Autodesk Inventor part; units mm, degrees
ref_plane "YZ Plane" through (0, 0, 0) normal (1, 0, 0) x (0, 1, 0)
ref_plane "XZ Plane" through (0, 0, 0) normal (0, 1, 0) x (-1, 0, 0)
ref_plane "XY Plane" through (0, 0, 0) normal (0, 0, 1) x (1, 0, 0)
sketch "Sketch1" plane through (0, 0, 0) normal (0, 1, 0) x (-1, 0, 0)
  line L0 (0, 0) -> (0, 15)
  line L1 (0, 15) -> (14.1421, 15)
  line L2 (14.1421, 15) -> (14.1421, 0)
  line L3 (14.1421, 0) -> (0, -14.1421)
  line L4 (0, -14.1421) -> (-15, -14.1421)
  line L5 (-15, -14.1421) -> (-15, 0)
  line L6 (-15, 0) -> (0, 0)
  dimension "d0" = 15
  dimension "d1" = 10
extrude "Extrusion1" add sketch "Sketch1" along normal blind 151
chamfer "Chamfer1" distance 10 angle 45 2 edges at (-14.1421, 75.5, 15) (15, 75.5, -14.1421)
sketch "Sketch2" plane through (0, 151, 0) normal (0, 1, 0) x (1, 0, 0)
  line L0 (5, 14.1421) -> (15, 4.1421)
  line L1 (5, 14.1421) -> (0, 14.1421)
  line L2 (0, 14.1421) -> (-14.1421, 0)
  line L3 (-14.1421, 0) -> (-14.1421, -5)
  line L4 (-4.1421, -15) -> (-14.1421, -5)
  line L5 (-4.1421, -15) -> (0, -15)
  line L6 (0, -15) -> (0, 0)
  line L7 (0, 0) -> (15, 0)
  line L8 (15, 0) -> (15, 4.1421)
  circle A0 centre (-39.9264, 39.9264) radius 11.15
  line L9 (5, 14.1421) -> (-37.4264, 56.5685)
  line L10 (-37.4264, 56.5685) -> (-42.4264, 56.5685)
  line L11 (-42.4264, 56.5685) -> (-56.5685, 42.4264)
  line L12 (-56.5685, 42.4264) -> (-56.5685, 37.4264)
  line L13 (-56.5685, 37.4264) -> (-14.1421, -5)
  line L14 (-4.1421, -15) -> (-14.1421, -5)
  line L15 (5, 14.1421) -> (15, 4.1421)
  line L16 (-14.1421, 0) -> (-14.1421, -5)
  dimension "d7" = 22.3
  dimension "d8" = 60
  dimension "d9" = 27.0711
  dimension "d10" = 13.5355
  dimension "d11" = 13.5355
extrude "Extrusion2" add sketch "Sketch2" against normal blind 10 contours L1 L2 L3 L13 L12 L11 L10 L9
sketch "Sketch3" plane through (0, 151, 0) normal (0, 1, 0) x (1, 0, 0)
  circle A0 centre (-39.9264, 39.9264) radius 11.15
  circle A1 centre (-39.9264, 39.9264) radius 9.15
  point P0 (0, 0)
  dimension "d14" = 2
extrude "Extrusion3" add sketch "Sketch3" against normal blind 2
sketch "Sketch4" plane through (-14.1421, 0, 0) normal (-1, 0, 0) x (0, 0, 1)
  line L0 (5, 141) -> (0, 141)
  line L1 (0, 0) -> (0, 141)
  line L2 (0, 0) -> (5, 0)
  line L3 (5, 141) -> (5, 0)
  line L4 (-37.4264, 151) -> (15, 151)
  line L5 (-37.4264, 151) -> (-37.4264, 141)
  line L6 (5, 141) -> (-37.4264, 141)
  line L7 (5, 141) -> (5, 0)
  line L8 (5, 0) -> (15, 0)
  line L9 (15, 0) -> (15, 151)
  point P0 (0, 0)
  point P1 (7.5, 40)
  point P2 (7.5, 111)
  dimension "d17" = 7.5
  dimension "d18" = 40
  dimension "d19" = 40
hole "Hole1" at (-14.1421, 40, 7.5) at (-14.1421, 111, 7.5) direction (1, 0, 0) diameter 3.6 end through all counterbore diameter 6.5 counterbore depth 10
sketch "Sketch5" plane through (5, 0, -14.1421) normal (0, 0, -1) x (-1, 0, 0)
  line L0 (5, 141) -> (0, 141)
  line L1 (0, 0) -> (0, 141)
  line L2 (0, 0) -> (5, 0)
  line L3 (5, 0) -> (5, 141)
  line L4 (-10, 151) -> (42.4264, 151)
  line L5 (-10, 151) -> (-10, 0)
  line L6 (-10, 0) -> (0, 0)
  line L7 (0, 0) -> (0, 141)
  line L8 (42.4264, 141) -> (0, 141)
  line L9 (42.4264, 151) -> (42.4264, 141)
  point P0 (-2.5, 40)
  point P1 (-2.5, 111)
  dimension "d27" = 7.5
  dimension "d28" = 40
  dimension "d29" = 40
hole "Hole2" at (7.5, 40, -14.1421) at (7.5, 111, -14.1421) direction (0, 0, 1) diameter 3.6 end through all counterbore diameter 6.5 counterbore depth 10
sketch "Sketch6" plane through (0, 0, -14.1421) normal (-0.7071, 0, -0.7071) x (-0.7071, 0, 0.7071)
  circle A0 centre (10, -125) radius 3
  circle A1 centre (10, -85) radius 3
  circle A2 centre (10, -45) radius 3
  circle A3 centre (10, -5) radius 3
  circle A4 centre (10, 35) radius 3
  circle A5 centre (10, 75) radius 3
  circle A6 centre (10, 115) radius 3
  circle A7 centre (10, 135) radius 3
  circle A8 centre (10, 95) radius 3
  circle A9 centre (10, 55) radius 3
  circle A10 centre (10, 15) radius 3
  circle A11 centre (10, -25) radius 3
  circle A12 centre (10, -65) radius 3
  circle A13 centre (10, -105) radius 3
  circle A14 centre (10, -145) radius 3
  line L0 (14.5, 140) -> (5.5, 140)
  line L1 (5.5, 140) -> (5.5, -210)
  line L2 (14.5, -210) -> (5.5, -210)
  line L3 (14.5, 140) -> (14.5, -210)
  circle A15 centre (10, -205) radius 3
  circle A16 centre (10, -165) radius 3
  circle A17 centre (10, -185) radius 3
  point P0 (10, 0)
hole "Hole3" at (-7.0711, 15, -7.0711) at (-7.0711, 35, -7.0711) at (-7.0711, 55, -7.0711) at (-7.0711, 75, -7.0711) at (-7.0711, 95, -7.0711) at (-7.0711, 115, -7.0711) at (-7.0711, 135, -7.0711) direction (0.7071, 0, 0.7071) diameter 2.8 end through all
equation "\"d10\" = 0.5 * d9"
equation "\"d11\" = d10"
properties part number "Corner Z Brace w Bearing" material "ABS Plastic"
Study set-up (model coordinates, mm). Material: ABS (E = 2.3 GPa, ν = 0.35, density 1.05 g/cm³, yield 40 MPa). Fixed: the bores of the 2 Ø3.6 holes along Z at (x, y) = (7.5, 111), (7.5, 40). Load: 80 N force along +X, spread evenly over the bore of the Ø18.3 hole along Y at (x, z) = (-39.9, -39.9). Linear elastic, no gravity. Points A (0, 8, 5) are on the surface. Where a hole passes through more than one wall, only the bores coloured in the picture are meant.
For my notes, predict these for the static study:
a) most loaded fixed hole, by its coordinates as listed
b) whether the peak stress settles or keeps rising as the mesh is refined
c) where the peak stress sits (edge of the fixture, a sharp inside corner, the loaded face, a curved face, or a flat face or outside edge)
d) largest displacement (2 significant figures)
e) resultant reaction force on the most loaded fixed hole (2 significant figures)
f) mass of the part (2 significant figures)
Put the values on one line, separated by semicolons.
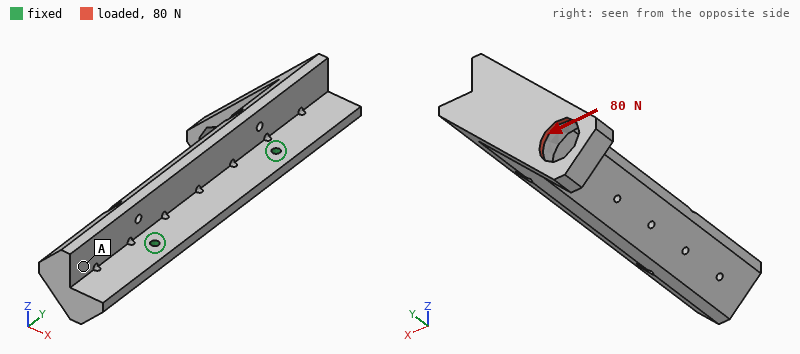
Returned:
(7.5, 111); keeps rising; edge of the fixture; 1.9 mm; 150 N; 79 g
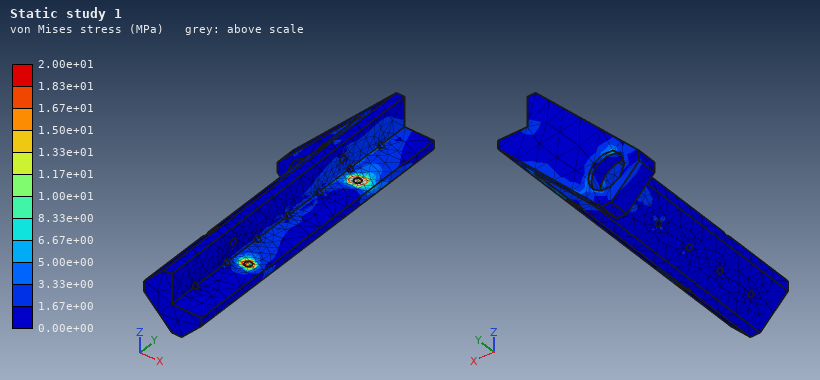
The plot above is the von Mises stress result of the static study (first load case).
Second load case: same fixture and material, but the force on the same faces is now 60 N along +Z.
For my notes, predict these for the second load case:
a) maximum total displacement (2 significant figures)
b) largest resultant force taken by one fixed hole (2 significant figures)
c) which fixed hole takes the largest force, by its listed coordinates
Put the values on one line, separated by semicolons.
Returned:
1.8 mm; 92 N; (7.5, 111)
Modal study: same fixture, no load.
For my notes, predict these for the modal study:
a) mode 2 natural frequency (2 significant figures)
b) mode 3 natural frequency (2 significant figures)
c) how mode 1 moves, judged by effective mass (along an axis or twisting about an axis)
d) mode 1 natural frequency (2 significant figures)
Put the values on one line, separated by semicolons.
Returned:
500 Hz; 940 Hz; along Z; 330 Hz
